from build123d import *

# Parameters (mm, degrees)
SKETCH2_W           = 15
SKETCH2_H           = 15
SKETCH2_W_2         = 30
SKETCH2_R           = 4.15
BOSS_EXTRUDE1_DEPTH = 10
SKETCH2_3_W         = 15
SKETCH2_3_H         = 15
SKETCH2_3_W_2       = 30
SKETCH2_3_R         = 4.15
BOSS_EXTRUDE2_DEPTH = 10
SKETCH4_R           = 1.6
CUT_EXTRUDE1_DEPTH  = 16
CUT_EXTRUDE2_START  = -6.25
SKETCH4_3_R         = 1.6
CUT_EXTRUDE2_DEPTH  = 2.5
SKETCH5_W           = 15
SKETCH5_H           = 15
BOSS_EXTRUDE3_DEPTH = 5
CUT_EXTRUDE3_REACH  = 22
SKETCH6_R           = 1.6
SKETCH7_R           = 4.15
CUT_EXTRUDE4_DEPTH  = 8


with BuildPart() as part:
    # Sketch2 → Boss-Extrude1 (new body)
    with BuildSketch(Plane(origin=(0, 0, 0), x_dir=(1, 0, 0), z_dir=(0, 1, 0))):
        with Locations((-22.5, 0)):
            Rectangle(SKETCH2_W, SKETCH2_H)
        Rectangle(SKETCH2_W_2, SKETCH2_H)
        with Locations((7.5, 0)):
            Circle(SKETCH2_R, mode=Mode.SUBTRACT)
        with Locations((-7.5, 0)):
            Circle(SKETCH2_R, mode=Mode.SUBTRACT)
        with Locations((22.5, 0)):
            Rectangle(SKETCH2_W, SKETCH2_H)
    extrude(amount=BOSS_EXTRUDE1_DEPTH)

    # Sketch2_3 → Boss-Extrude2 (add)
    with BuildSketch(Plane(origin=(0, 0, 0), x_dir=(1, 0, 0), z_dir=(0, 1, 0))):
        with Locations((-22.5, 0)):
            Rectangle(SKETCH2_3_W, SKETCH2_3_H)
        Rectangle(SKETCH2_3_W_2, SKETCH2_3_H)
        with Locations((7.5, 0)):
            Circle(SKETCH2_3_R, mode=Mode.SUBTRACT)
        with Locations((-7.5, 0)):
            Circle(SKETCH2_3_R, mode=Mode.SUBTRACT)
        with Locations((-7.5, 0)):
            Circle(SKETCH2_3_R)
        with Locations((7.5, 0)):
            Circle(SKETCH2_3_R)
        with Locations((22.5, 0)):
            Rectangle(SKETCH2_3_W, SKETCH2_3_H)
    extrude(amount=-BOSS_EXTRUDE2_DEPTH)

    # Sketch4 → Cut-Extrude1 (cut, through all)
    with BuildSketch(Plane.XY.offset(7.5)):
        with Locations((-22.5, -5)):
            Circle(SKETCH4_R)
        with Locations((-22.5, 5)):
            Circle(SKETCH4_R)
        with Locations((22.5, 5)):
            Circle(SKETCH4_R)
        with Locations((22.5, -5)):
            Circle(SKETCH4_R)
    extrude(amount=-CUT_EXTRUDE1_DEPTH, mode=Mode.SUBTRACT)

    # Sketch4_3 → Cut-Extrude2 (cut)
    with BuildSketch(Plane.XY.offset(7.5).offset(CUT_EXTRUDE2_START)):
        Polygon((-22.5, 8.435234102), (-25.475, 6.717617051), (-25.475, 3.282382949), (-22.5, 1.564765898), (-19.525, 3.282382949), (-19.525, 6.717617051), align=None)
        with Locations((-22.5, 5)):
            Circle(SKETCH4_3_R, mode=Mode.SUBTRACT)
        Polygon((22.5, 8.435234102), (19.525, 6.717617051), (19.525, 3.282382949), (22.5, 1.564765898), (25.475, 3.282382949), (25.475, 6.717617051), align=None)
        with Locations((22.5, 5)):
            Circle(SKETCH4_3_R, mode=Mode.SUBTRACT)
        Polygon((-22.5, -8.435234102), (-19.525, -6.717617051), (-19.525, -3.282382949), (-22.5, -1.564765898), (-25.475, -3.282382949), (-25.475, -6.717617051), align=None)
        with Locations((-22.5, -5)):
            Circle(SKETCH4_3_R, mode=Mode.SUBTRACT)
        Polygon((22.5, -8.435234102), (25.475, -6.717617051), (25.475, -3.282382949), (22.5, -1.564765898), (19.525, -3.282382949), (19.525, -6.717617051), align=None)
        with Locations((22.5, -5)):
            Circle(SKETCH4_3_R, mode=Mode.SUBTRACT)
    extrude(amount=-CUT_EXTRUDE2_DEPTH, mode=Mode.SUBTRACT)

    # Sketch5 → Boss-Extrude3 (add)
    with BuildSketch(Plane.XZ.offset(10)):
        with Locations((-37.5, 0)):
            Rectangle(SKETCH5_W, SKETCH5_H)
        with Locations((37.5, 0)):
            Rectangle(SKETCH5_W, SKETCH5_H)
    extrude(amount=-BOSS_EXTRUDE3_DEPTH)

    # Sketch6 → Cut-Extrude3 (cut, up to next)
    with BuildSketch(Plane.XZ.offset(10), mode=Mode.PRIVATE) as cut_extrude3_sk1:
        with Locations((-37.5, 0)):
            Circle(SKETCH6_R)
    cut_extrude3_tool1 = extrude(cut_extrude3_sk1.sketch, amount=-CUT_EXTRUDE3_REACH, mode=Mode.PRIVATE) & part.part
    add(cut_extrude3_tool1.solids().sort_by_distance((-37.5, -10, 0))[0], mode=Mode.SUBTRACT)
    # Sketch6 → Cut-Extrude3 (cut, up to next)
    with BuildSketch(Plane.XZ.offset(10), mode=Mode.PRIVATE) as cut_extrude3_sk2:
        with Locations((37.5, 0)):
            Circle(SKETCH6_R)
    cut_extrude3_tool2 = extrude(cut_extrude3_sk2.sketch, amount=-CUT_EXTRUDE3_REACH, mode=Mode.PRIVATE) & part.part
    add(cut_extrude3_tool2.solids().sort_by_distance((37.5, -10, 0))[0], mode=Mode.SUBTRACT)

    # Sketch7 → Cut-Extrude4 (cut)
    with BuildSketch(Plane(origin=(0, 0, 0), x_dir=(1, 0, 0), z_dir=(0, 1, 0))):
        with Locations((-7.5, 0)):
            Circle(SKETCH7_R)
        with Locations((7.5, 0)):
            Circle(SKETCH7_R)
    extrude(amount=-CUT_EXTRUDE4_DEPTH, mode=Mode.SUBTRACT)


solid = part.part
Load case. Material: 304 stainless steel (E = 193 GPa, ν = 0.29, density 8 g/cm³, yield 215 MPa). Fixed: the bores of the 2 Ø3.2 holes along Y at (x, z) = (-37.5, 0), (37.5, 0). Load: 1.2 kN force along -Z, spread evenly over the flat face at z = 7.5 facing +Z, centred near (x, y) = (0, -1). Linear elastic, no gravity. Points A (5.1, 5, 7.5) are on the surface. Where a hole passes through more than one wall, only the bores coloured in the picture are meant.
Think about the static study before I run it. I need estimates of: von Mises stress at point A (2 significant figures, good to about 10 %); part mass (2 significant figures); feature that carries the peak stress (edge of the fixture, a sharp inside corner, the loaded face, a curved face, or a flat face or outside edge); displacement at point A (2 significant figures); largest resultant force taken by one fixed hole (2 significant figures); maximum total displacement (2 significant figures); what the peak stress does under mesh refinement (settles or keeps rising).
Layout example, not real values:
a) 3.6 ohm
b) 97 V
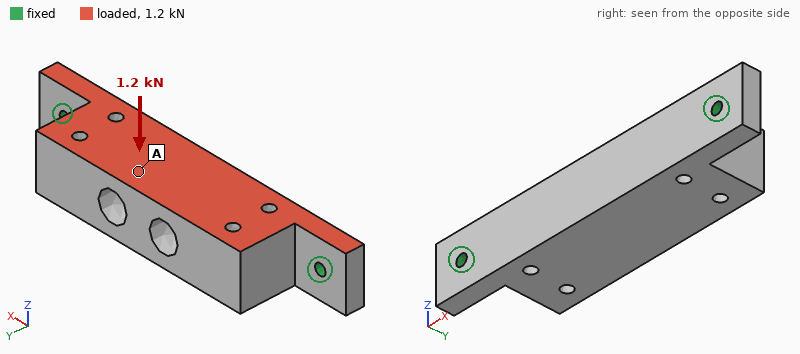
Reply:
a) 14 MPa
b) 140 g
c) edge of the fixture
d) 19 µm
e) 600 N
f) 23 µm
g) keeps rising
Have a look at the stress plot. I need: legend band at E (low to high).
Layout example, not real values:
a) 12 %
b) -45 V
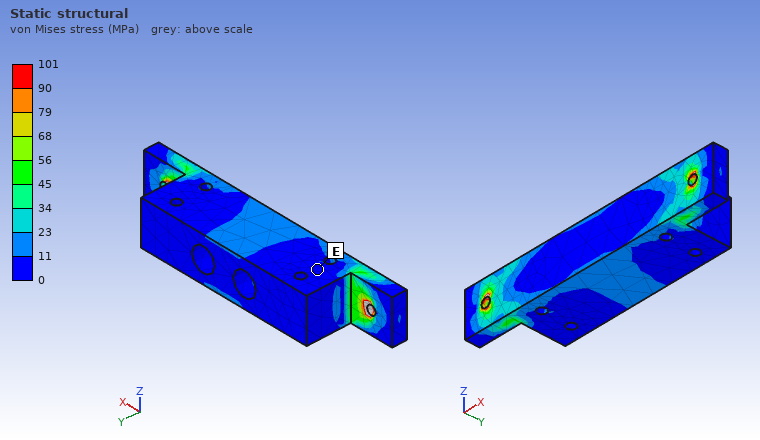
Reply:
a) 0 to 11 MPa
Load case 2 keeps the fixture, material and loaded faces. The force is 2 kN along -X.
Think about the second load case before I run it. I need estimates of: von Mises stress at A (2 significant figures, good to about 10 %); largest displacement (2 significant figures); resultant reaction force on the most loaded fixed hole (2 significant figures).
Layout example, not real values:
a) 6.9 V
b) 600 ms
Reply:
a) 5.6 MPa
b) 2.8 µm
c) 1.0 kN
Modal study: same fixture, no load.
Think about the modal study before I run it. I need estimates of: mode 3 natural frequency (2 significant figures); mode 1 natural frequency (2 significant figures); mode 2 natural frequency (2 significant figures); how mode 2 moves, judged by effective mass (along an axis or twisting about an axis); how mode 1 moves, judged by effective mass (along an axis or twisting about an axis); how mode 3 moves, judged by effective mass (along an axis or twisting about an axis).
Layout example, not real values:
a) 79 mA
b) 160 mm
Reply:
a) 9100 Hz
b) 3700 Hz
c) 7000 Hz
d) along Y
e) along Z
f) along Z
